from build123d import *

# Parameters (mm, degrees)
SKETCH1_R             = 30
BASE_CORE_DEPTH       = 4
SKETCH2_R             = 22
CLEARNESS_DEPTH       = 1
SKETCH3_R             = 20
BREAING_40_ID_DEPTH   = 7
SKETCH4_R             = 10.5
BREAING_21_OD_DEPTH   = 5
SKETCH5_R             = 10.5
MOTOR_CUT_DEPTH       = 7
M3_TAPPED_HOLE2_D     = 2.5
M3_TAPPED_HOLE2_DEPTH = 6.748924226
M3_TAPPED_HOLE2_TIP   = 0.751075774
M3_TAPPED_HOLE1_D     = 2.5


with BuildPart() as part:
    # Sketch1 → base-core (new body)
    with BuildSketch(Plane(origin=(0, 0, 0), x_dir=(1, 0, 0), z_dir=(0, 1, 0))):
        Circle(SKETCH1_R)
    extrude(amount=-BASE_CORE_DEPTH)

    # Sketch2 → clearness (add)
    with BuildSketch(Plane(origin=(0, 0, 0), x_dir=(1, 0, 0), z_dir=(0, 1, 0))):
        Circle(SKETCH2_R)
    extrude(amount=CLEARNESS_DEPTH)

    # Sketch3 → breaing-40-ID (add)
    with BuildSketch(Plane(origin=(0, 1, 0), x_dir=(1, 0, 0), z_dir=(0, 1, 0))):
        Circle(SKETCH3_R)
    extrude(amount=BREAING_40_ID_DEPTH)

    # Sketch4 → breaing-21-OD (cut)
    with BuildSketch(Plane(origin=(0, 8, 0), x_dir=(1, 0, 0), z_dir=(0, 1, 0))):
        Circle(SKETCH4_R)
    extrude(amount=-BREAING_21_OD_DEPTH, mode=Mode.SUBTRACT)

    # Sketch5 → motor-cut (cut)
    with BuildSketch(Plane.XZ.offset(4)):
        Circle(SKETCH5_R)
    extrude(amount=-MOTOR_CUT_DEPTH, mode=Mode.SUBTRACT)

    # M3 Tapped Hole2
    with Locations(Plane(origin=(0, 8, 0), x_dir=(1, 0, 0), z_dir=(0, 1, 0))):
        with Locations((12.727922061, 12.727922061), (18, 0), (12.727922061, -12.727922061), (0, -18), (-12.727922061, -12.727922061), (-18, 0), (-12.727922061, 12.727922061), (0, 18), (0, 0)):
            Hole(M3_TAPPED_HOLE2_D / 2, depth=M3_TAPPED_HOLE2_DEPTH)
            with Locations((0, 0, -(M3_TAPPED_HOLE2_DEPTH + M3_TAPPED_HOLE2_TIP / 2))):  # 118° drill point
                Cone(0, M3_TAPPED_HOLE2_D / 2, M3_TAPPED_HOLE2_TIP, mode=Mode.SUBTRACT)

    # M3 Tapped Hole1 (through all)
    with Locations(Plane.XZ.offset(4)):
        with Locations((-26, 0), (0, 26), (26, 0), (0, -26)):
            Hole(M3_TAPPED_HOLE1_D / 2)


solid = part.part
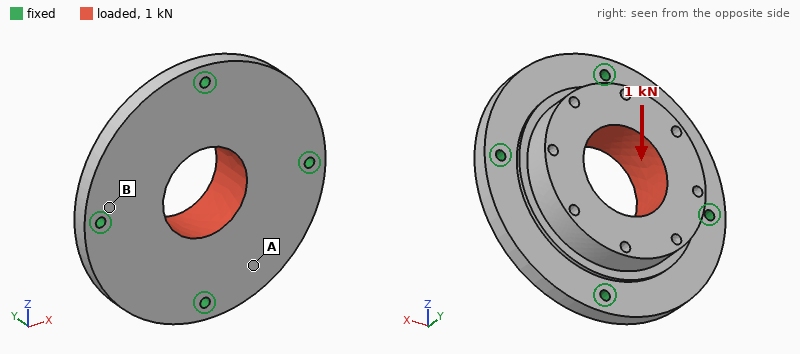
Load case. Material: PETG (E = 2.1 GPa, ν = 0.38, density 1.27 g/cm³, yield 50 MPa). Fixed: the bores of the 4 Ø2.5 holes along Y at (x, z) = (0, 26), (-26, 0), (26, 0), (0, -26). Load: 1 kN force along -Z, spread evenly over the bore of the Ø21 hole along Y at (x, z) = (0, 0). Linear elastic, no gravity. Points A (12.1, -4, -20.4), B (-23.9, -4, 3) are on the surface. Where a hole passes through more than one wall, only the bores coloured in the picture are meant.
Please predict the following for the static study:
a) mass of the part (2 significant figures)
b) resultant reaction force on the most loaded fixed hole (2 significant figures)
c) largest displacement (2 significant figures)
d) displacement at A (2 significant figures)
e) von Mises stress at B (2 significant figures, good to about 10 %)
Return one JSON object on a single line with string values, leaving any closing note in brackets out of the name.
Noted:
{"mass of the part": "22 g", "resultant reaction force on the most loaded fixed hole": "310 N", "largest displacement": "57 µm", "displacement at A": "36 µm", "von Mises stress at B": "4.2 MPa"}
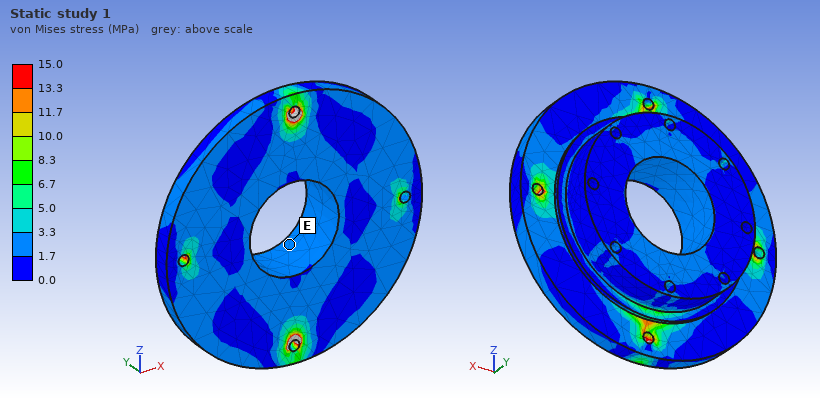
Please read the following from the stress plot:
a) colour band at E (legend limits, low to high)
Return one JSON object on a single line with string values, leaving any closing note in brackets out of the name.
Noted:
{"colour band at E": "1.7 to 3.3 MPa"}
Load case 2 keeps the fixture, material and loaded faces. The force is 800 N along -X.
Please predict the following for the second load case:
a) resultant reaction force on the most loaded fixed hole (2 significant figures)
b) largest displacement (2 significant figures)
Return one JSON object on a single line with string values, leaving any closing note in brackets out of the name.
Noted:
{"resultant reaction force on the most loaded fixed hole": "250 N", "largest displacement": "45 µm"}
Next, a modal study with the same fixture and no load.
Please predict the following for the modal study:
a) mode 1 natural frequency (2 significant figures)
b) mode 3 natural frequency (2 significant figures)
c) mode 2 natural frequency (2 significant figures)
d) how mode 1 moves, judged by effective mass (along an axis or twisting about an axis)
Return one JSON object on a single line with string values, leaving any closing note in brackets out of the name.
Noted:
{"mode 1 natural frequency": "3200 Hz", "mode 3 natural frequency": "3700 Hz", "mode 2 natural frequency": "3700 Hz", "how mode 1 moves, judged by effective mass": "along Y"}
